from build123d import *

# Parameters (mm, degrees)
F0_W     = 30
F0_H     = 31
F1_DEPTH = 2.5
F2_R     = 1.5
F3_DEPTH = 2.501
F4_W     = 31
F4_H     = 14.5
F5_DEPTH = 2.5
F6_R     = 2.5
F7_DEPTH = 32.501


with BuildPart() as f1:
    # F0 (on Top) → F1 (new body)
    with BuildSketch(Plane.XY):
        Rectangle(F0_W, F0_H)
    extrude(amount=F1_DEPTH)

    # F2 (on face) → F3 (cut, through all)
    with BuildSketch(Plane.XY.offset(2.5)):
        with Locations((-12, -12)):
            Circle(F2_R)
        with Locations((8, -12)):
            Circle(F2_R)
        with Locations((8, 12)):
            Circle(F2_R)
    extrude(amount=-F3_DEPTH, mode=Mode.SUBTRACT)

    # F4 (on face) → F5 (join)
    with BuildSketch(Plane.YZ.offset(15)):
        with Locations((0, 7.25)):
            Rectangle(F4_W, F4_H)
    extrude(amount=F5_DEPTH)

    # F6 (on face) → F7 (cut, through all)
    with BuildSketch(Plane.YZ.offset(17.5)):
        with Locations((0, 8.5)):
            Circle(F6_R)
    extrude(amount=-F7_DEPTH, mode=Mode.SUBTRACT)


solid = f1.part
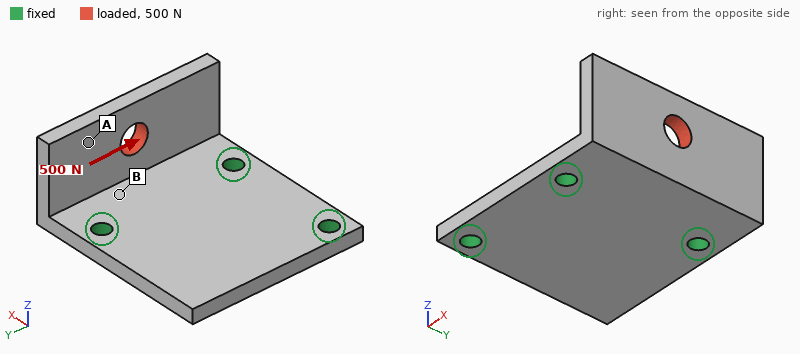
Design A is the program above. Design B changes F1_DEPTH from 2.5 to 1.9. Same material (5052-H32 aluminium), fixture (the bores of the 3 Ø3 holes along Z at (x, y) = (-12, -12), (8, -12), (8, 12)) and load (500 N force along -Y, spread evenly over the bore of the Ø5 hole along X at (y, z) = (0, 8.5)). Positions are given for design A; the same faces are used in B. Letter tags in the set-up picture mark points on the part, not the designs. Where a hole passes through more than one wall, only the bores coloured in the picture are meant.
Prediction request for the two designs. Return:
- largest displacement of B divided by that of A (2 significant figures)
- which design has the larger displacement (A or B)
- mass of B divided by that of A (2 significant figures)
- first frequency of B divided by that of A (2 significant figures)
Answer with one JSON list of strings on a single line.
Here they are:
["1.7", "B", "0.84", "0.70"]
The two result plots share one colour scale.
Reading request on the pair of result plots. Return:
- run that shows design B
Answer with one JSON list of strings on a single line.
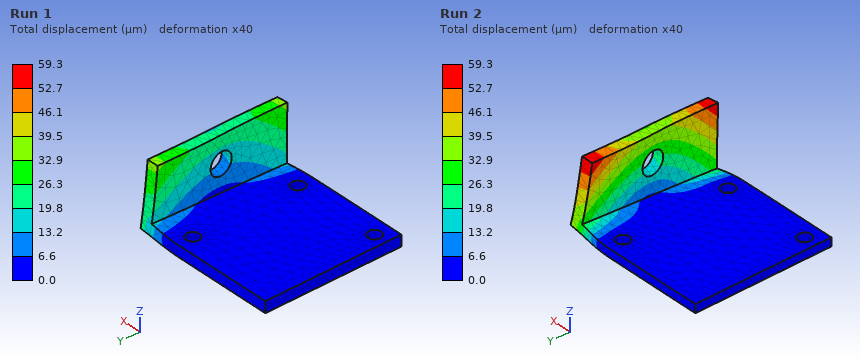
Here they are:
["Run 2"]
